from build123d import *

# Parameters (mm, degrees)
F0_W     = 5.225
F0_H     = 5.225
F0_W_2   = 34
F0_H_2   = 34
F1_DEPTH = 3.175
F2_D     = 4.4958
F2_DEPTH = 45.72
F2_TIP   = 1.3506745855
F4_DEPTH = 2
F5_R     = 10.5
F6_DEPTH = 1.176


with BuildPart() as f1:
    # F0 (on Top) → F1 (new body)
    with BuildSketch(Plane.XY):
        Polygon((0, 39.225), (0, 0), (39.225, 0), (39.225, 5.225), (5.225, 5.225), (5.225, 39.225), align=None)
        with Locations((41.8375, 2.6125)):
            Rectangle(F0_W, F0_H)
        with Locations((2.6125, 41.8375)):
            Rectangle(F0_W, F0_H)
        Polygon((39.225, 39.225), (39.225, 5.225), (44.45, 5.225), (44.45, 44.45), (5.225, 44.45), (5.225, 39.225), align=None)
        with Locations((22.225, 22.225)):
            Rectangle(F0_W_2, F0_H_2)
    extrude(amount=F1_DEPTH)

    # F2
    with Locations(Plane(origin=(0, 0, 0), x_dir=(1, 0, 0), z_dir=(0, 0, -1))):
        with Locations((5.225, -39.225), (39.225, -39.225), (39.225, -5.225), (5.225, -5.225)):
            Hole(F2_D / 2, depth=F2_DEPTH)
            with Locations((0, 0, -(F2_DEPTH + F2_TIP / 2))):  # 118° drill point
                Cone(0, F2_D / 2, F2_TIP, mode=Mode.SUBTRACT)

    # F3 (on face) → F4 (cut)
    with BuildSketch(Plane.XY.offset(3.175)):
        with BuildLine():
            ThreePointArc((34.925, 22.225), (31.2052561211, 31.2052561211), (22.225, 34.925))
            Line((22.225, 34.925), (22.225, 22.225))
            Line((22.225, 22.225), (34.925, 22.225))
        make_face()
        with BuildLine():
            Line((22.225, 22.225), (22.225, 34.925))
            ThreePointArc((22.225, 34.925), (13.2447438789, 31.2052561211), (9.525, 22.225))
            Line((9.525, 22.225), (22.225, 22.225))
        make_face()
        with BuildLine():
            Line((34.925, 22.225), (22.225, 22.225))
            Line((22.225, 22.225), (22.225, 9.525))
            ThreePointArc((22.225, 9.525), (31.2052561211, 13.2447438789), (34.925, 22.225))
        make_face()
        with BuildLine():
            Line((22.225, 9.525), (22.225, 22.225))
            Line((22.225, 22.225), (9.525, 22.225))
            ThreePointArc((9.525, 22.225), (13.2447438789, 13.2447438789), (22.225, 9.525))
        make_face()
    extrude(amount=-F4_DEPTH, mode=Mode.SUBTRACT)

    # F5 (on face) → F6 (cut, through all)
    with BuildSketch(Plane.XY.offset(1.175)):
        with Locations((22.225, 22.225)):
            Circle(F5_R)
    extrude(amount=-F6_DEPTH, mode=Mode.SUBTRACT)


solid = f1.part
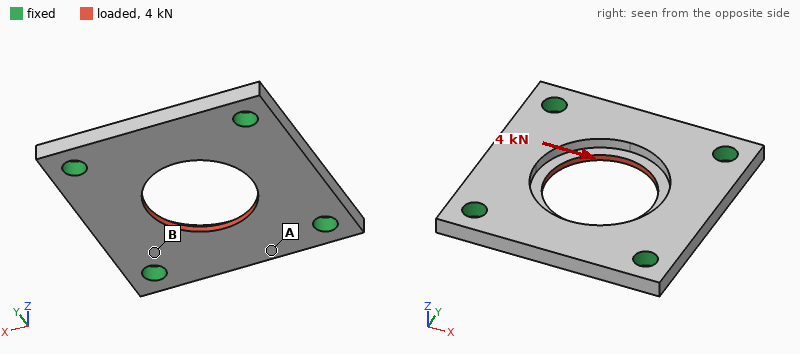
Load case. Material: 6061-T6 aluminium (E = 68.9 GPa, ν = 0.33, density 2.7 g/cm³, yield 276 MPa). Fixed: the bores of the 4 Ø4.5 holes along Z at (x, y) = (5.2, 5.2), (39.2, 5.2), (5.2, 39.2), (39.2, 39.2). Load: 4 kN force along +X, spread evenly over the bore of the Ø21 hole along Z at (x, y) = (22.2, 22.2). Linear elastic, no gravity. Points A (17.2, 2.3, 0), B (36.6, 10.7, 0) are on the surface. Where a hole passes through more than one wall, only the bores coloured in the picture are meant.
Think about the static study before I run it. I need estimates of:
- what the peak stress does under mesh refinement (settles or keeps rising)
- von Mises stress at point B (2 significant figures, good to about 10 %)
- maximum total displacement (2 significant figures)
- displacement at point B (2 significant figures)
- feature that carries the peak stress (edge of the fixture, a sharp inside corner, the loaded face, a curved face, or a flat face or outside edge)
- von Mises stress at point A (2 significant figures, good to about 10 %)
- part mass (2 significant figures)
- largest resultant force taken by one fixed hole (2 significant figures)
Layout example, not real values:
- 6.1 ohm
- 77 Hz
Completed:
- keeps rising
- 44 MPa
- 22 µm
- 4.7 µm
- edge of the fixture
- 11 MPa
- 13 g
- 1.1 kN
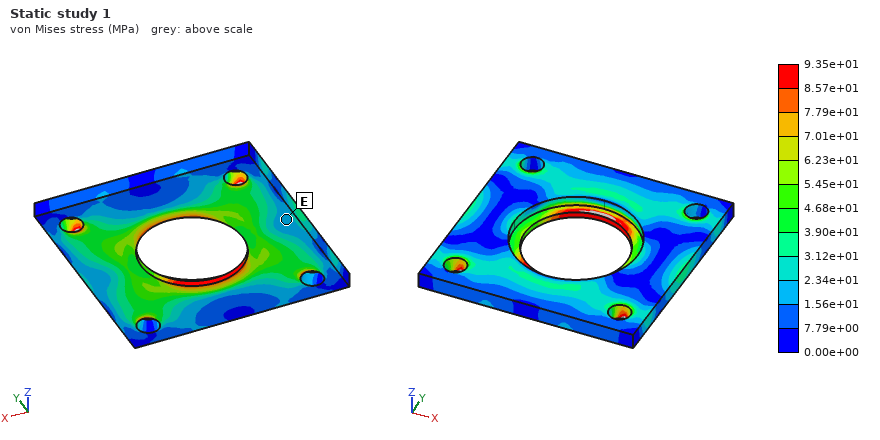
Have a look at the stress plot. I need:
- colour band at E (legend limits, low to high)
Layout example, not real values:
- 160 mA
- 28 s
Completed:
- 1.56e+01 to 2.34e+01 MPa
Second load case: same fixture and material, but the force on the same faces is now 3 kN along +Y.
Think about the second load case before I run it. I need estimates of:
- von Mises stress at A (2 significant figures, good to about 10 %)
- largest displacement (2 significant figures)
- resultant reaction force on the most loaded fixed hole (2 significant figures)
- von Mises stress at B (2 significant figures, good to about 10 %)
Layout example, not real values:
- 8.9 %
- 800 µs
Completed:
- 17 MPa
- 16 µm
- 790 N
- 25 MPa
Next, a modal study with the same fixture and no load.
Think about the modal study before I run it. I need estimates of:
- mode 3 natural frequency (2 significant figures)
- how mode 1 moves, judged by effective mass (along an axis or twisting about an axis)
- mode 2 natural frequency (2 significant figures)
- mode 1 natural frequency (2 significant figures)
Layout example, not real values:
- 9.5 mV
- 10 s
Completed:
- 16 kHz
- along Z
- 16 kHz
- 15 kHz
